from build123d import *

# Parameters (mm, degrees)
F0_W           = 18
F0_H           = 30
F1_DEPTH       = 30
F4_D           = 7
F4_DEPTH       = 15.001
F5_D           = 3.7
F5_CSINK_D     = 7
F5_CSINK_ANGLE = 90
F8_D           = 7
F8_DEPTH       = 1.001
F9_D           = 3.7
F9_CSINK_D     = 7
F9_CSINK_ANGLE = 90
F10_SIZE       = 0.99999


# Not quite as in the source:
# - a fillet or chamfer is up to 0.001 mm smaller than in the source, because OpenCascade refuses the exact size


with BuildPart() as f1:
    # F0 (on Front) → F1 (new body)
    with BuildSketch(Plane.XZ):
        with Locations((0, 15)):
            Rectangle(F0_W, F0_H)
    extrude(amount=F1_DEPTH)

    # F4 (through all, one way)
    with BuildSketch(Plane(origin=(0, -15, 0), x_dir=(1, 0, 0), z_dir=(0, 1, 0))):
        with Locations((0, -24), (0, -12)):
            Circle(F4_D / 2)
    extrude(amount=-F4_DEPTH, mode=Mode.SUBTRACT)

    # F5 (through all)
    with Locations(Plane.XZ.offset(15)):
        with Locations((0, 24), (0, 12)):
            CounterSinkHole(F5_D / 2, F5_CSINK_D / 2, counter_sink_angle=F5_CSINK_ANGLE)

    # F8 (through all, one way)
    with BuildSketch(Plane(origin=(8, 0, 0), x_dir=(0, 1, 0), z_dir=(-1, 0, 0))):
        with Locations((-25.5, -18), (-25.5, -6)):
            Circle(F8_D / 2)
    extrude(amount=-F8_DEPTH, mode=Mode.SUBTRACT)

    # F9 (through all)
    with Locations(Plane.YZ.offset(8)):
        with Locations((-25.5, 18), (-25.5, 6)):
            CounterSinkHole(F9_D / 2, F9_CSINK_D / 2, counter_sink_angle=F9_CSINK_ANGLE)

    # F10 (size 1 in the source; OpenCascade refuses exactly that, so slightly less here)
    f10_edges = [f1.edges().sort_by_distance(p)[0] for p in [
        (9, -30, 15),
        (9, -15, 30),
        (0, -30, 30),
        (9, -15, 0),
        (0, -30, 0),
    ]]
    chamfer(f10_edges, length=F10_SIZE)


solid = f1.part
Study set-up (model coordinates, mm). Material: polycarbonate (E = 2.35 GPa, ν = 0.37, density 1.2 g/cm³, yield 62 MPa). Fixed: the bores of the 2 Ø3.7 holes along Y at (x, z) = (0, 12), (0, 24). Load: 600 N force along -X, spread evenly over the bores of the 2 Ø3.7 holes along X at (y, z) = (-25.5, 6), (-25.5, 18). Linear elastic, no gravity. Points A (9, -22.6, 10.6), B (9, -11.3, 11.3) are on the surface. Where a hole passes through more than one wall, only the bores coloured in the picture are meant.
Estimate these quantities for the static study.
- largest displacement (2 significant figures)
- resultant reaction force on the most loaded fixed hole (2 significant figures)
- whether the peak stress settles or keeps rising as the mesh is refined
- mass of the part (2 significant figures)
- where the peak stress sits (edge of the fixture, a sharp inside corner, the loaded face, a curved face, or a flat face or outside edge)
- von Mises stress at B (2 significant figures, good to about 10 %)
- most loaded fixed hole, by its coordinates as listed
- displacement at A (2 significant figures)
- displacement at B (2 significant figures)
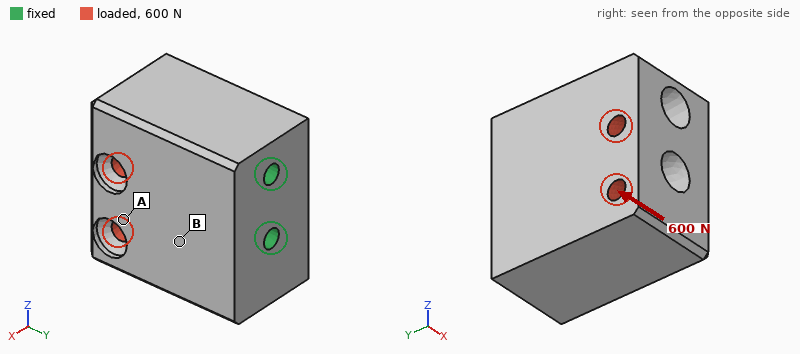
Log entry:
0.19 mm
540 N
keeps rising
17 g
edge of the fixture
7.1 MPa
(0, 12)
0.12 mm
0.045 mm
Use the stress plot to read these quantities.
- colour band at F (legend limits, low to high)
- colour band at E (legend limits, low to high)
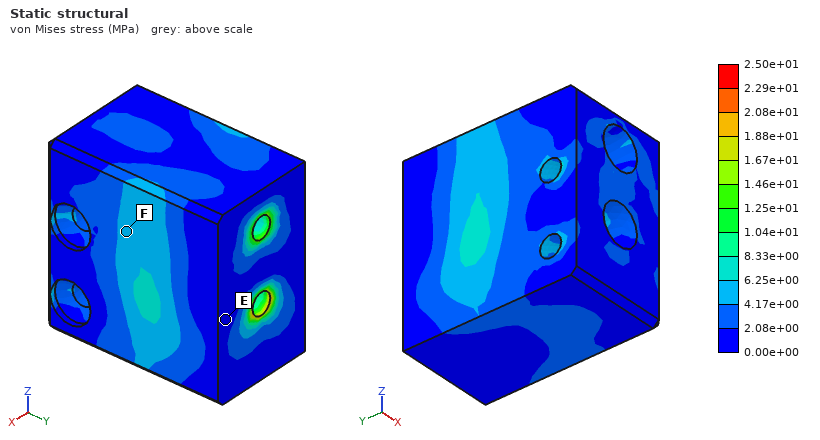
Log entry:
4.17e+00 to 6.25e+00 MPa
0.00e+00 to 2.08e+00 MPa
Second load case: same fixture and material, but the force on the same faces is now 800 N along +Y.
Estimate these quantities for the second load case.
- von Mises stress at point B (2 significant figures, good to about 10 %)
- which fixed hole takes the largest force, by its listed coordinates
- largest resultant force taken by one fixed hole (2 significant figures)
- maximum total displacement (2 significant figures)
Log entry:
1.2 MPa
(0, 12)
630 N
54 µm
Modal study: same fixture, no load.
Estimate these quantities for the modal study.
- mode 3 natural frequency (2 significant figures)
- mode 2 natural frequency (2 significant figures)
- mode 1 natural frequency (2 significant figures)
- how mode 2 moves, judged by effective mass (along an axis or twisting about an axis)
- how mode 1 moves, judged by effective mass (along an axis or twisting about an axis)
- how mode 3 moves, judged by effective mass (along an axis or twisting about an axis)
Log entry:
6600 Hz
5600 Hz
4500 Hz
along Z
along X
twisting about Y
